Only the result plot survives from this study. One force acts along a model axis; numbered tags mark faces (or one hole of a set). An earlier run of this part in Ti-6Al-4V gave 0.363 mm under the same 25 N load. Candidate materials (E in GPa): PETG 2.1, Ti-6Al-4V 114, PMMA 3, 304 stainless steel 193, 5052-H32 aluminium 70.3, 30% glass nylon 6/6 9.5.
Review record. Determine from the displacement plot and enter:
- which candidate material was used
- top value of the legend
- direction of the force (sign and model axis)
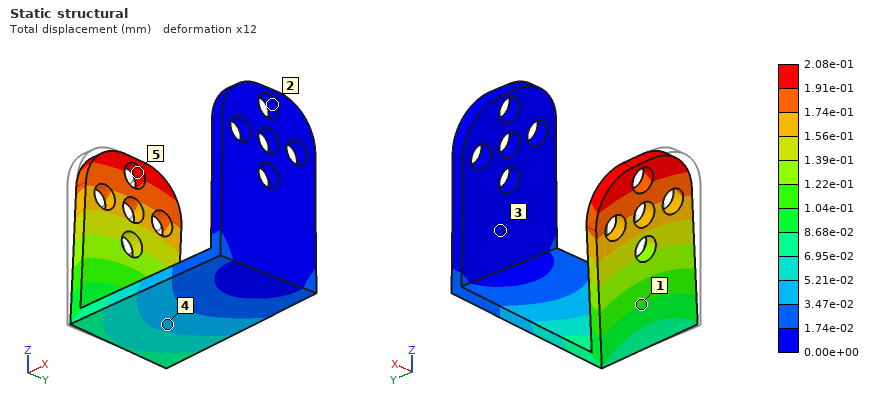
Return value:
304 stainless steel
2.08e-01 mm
+Y
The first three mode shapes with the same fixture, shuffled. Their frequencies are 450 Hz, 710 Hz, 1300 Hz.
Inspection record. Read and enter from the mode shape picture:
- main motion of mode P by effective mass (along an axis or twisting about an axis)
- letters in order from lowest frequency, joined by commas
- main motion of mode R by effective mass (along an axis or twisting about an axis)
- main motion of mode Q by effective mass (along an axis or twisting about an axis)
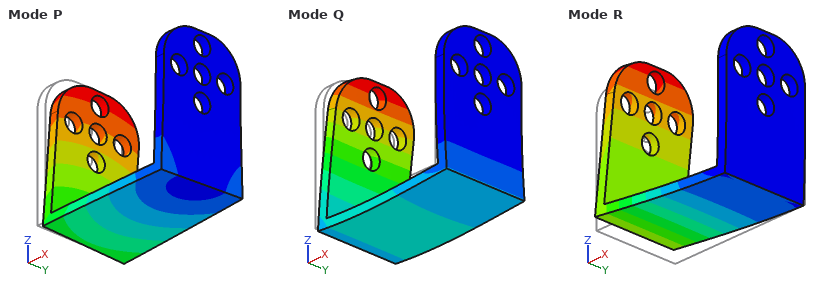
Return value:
along Y
R, P, Q
along Z
along X
